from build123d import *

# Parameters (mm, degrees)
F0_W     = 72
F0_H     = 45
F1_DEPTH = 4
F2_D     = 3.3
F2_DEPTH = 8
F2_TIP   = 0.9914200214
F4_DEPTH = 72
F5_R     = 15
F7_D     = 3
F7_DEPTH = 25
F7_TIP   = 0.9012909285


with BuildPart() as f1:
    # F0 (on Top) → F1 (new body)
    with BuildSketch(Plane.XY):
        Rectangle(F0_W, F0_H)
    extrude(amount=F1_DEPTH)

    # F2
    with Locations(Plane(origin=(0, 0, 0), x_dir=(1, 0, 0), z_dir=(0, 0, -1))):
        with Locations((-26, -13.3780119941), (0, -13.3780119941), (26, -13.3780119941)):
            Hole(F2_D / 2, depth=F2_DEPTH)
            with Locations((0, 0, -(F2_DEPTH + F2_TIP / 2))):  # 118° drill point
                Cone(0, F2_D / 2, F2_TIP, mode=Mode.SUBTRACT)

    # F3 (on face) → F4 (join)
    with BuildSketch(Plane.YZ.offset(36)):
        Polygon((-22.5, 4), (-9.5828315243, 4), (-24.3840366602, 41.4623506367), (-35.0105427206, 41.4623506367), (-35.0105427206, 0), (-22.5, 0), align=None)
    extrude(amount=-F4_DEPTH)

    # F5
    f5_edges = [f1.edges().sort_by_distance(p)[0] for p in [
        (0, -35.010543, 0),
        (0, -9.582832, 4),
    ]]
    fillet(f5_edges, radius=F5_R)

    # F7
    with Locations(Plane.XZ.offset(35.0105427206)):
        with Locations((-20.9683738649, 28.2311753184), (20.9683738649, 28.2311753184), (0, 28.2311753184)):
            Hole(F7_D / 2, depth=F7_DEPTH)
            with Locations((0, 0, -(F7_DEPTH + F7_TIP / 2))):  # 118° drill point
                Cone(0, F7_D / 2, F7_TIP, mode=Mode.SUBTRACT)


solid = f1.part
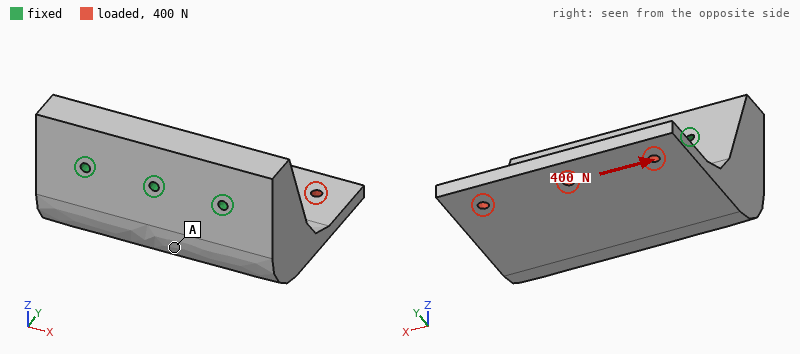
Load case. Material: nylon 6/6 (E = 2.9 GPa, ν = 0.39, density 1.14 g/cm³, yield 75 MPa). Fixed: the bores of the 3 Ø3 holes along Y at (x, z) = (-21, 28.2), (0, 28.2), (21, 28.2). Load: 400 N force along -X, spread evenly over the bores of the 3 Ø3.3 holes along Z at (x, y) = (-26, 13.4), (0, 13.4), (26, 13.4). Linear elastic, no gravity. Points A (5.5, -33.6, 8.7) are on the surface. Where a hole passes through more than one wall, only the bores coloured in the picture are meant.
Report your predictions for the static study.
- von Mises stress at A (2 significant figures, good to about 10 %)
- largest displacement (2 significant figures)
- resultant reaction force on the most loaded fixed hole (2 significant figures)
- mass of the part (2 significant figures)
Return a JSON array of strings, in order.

["1.1 MPa", "0.20 mm", "400 N", "71 g"]
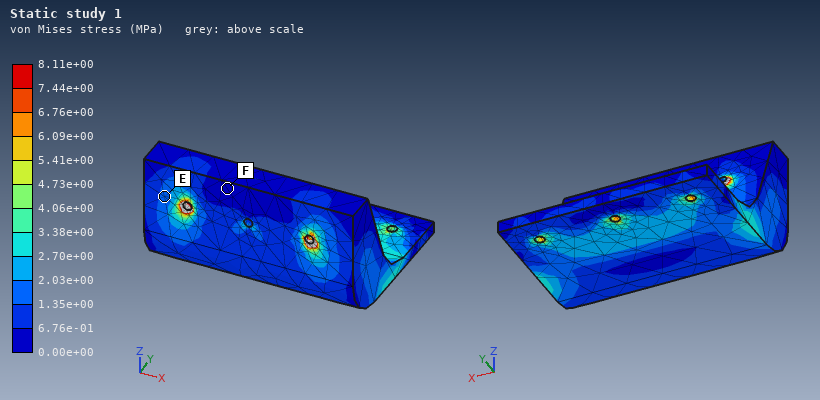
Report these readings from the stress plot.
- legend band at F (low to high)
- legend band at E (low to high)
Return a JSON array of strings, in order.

["0.00e+00 to 6.76e-01 MPa", "1.35e+00 to 2.03e+00 MPa"]
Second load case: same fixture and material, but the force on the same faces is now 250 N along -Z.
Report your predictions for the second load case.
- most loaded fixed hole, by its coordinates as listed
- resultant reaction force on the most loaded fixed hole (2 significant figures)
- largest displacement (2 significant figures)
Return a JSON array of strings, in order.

["(0, 28.2)", "120 N", "1.1 mm"]
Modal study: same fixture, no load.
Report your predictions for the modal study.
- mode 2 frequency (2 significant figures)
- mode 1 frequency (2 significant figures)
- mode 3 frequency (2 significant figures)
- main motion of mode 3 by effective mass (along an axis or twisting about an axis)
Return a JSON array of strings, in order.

["1500 Hz", "1100 Hz", "2400 Hz", "along Y"]
